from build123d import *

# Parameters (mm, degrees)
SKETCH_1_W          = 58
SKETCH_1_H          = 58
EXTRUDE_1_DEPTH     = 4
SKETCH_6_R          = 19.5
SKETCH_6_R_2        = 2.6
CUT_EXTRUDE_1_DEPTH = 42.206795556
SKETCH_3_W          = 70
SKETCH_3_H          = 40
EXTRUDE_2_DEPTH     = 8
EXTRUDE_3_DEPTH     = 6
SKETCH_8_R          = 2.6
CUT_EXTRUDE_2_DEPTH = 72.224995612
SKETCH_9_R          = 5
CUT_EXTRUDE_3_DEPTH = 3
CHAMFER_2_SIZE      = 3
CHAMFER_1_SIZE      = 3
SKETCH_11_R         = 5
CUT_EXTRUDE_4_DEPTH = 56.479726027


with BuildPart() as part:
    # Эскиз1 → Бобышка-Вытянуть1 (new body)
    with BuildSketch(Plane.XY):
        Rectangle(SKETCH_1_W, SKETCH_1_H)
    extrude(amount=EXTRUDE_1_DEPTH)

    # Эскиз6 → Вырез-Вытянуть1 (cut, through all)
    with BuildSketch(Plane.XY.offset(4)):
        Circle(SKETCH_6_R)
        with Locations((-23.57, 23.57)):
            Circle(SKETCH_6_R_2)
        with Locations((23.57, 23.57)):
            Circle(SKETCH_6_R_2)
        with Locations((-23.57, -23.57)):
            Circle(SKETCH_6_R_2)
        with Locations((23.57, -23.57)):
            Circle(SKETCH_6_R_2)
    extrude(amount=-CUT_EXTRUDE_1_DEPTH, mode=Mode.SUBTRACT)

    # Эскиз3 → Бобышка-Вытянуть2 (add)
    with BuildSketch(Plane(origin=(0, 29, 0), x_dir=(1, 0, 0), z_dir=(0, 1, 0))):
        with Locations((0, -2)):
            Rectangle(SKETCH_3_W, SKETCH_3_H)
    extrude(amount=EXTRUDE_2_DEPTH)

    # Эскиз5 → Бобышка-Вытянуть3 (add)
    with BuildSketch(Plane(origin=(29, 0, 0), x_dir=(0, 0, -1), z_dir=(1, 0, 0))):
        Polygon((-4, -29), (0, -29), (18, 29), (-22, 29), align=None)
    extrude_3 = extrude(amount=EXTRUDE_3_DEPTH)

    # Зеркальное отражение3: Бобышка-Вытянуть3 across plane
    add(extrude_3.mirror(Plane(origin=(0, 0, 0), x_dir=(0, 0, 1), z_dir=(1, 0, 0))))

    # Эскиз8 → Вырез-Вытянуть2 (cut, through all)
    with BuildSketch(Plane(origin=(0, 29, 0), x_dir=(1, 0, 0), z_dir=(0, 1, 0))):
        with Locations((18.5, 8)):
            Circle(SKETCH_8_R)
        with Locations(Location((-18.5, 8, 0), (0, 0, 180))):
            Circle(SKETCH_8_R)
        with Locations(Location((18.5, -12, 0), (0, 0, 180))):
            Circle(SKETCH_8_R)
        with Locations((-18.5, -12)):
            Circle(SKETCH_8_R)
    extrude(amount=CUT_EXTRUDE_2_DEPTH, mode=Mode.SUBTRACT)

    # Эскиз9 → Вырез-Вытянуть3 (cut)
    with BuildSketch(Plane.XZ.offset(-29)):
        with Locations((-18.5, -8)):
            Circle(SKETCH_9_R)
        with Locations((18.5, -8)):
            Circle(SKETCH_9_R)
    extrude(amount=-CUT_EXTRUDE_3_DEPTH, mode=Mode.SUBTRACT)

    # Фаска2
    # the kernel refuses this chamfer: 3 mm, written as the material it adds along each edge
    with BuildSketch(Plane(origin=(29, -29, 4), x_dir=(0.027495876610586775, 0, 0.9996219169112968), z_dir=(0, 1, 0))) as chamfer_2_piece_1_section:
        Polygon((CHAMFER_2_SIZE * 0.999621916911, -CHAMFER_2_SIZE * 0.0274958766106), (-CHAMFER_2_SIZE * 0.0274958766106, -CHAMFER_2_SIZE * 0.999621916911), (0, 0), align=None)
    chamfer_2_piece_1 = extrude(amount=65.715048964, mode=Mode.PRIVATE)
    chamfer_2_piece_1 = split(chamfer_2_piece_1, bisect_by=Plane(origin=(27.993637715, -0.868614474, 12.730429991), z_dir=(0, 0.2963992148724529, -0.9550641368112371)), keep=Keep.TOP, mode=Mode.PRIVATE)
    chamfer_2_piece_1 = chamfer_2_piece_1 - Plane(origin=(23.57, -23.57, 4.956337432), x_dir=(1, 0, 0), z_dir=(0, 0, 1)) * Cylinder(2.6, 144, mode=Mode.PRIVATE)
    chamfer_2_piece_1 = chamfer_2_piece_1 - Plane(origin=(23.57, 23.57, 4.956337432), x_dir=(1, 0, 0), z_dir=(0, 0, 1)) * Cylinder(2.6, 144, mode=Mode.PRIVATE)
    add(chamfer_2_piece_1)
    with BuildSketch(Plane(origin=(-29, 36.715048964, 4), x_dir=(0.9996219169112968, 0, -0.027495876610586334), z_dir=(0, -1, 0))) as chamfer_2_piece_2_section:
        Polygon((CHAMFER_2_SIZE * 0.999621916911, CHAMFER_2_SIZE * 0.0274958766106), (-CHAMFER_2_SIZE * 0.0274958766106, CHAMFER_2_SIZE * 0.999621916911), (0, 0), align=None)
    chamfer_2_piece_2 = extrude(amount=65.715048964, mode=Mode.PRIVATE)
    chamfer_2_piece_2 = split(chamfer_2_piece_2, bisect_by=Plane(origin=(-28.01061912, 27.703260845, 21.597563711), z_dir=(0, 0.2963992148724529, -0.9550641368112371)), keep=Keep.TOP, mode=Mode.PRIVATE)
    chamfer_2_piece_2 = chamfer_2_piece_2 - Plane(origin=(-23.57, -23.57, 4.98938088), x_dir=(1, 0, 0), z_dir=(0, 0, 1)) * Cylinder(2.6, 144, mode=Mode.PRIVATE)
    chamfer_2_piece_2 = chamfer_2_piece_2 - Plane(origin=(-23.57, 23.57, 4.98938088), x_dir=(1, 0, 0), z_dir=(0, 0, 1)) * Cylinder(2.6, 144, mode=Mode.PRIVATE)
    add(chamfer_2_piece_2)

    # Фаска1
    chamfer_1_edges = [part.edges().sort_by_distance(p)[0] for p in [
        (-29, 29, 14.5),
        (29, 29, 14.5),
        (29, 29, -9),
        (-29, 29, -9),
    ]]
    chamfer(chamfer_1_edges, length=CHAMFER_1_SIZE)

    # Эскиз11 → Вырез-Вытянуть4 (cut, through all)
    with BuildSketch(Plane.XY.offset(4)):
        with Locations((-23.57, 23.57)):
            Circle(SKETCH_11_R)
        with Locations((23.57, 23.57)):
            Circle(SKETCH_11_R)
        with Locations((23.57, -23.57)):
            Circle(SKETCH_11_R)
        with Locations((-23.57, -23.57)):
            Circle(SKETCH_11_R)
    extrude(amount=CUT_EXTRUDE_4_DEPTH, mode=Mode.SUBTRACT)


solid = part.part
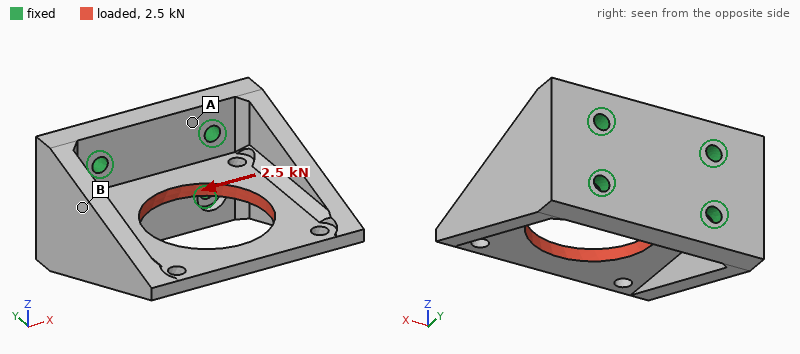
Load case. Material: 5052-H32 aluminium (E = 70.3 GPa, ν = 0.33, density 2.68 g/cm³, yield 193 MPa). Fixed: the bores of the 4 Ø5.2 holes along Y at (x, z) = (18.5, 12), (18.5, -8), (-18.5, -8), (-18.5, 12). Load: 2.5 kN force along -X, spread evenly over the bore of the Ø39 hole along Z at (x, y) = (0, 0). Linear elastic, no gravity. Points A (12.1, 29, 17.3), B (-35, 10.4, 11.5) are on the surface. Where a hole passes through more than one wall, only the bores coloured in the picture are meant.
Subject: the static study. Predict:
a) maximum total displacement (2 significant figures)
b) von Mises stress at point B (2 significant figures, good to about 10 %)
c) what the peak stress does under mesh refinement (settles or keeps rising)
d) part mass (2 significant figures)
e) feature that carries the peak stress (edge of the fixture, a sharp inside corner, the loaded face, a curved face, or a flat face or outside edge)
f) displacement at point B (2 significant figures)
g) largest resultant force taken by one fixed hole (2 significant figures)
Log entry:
75 µm
9.8 MPa
keeps rising
120 g
edge of the fixture
29 µm
1.2 kN
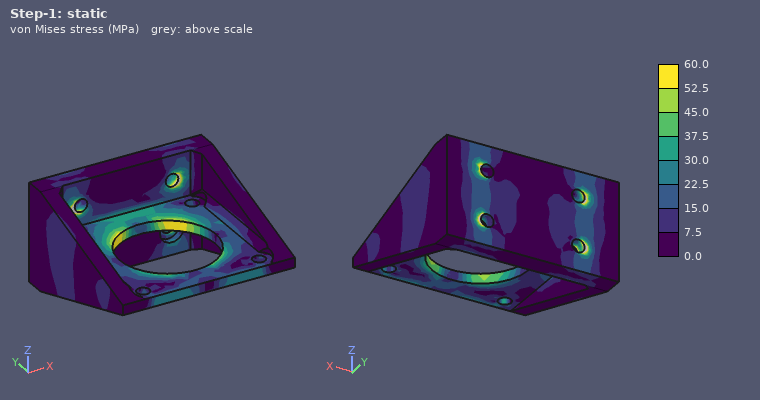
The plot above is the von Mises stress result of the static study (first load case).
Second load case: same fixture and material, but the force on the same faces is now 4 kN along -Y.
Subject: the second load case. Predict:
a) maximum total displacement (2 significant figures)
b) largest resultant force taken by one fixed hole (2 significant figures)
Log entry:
36 µm
1.1 kN
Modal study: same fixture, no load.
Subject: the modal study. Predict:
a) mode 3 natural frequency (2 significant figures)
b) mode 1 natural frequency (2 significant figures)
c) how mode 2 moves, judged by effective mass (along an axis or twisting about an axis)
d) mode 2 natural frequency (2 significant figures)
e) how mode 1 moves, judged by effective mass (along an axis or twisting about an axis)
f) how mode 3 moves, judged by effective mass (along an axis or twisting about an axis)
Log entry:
4900 Hz
3300 Hz
along X
4500 Hz
along Z
along X
